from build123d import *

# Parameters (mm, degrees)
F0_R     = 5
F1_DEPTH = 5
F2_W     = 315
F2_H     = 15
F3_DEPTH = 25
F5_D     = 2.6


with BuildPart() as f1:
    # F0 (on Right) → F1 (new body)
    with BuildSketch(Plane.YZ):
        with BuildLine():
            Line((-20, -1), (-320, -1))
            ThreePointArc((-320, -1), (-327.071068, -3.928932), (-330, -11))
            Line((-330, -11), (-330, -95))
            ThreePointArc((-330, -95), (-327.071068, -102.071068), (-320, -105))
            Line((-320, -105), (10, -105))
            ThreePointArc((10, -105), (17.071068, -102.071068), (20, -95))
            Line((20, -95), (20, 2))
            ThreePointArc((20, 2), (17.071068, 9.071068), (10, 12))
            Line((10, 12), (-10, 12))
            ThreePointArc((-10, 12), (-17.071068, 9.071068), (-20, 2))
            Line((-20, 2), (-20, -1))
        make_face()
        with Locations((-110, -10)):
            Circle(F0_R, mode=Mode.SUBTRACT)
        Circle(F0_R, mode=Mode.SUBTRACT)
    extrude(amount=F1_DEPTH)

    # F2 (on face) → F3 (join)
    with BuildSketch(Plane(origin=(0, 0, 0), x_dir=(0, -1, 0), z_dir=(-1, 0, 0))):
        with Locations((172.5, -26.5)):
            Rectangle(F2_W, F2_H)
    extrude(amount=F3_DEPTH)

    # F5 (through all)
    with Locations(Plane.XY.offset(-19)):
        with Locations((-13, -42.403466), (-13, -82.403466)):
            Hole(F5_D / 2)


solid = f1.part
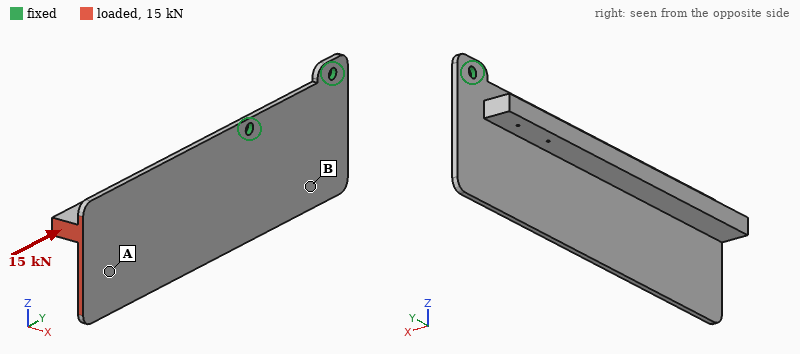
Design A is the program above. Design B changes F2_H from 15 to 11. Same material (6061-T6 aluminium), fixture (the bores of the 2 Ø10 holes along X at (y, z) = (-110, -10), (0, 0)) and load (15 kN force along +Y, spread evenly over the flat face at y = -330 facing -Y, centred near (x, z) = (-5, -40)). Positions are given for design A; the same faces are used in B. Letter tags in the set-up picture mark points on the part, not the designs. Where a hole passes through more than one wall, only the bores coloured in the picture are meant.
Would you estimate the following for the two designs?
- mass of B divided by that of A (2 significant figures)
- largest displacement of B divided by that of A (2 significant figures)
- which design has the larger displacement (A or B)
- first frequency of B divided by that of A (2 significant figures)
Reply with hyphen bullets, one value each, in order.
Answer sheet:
- 0.90
- 1.1
- B
- 0.91
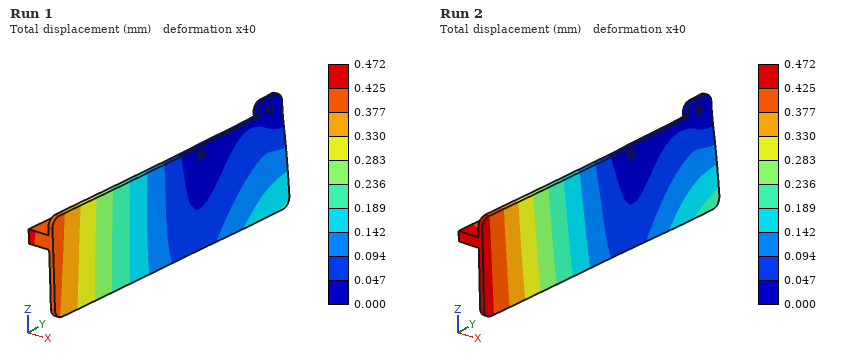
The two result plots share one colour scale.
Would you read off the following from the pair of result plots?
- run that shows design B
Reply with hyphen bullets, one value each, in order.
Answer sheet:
- Run 2
